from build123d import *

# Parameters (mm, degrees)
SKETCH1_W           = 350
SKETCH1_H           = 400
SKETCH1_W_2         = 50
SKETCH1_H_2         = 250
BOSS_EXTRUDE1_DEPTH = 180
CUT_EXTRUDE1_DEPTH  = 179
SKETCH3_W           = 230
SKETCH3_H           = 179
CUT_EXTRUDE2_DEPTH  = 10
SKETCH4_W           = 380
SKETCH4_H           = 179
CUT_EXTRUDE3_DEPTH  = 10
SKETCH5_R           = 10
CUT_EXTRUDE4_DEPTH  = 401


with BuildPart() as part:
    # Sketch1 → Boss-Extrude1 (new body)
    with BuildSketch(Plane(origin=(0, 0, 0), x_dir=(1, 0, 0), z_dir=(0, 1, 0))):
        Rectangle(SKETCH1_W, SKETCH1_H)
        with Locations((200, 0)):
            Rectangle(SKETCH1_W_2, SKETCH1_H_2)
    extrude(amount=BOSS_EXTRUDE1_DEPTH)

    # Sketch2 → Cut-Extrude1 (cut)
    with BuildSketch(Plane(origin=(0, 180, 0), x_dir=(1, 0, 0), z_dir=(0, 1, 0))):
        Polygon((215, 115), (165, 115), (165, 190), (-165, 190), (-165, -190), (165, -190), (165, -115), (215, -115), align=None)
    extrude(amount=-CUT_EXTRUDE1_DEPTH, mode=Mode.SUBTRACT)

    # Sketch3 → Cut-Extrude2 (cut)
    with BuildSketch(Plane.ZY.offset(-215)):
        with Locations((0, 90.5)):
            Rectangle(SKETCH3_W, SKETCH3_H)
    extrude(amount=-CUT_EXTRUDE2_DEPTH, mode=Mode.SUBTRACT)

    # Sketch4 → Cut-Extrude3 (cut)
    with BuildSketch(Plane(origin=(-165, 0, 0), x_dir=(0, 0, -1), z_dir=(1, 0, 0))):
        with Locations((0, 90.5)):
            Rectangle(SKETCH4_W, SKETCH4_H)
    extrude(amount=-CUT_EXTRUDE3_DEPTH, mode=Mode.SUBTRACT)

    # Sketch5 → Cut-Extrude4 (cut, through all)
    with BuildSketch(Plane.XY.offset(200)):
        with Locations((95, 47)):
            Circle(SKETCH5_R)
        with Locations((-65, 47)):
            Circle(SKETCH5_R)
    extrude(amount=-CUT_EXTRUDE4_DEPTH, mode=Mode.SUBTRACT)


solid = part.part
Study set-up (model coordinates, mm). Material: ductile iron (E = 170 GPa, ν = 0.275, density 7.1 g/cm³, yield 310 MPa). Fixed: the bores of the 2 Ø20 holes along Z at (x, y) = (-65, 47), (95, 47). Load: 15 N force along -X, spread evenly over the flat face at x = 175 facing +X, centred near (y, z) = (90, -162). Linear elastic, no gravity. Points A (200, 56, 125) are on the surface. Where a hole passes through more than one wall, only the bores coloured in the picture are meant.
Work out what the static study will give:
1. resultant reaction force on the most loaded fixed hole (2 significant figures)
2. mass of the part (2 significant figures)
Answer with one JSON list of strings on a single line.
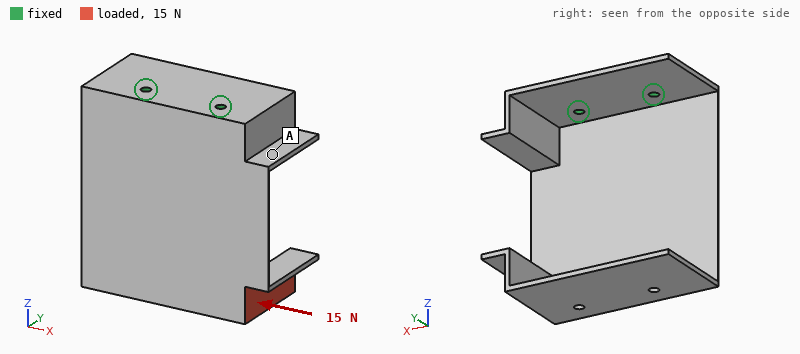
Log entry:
["30 N", "13 kg"]
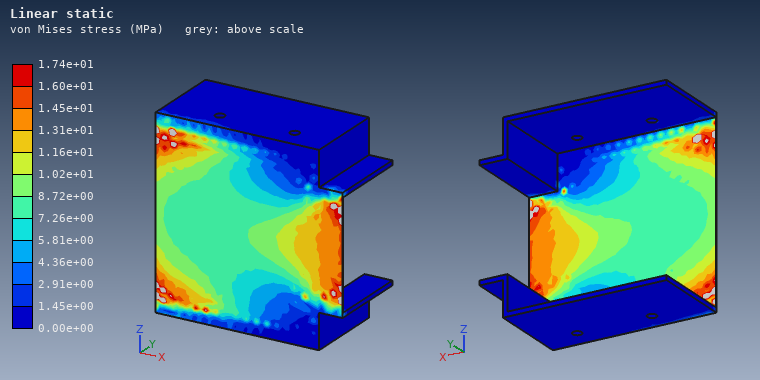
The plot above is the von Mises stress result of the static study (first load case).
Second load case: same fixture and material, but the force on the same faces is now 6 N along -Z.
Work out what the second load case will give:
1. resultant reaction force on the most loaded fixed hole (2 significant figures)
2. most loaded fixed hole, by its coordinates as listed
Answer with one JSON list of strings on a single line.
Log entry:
["7.6 N", "(95, 47)"]
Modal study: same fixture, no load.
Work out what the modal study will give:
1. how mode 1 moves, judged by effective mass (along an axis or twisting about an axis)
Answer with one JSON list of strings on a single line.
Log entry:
["along Y"]
